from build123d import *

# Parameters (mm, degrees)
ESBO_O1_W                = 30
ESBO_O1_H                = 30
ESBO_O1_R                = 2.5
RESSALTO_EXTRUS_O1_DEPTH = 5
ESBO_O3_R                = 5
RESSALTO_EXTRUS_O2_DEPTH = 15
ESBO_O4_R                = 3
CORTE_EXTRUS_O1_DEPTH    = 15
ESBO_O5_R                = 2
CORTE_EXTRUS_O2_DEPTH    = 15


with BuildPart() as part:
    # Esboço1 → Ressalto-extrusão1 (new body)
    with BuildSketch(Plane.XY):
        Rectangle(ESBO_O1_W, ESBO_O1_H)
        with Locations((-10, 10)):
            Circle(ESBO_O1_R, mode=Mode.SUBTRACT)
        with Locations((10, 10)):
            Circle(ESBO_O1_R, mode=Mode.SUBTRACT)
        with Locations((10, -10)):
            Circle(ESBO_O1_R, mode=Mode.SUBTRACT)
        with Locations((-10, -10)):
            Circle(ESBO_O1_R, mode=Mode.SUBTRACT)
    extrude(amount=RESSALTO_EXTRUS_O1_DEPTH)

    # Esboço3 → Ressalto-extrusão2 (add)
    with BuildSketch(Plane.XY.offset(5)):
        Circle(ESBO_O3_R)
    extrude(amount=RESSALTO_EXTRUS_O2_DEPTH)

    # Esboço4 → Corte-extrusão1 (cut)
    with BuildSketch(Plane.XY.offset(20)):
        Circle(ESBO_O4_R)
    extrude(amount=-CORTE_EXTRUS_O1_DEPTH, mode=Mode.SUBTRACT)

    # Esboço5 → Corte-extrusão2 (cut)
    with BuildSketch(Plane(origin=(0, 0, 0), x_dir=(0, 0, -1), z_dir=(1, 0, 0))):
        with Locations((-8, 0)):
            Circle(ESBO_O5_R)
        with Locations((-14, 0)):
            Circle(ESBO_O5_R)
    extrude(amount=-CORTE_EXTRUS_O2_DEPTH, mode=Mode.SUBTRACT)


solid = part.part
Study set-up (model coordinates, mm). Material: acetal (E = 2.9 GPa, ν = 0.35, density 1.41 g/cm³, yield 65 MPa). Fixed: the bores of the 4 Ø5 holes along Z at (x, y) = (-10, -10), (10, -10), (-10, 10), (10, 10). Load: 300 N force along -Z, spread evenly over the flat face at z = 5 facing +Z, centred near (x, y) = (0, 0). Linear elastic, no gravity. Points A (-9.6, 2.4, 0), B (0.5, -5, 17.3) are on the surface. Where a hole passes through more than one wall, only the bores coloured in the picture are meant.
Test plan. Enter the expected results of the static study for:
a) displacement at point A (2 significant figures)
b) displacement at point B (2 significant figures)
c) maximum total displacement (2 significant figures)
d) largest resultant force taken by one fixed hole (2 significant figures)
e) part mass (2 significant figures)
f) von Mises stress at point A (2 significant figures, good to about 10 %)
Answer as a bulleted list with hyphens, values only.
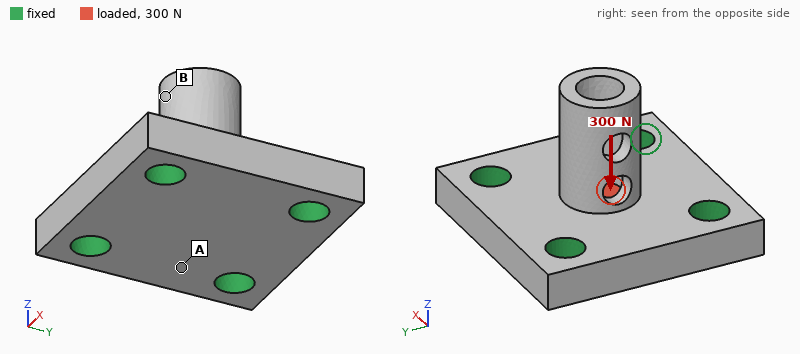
- 12 µm
- 30 µm
- 48 µm
- 76 N
- 6.8 g
- 2.5 MPa
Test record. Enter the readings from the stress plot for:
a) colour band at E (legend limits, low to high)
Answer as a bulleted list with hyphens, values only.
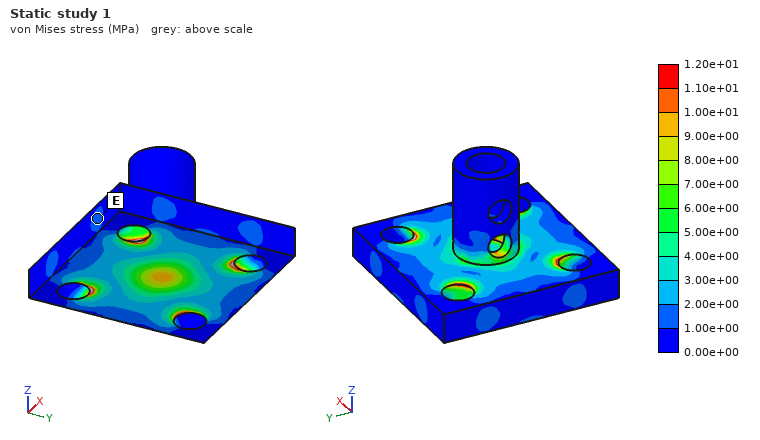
- 1.00e+00 to 2.00e+00 MPa
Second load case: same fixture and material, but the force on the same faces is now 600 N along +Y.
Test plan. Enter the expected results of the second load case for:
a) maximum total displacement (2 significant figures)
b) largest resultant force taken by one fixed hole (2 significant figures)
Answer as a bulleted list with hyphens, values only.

- 53 µm
- 170 N
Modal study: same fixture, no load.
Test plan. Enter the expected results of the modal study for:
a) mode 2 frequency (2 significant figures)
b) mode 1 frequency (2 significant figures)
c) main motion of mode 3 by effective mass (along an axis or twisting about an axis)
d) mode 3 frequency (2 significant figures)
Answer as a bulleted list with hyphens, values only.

- 5500 Hz
- 5300 Hz
- along Z
- 10 kHz
